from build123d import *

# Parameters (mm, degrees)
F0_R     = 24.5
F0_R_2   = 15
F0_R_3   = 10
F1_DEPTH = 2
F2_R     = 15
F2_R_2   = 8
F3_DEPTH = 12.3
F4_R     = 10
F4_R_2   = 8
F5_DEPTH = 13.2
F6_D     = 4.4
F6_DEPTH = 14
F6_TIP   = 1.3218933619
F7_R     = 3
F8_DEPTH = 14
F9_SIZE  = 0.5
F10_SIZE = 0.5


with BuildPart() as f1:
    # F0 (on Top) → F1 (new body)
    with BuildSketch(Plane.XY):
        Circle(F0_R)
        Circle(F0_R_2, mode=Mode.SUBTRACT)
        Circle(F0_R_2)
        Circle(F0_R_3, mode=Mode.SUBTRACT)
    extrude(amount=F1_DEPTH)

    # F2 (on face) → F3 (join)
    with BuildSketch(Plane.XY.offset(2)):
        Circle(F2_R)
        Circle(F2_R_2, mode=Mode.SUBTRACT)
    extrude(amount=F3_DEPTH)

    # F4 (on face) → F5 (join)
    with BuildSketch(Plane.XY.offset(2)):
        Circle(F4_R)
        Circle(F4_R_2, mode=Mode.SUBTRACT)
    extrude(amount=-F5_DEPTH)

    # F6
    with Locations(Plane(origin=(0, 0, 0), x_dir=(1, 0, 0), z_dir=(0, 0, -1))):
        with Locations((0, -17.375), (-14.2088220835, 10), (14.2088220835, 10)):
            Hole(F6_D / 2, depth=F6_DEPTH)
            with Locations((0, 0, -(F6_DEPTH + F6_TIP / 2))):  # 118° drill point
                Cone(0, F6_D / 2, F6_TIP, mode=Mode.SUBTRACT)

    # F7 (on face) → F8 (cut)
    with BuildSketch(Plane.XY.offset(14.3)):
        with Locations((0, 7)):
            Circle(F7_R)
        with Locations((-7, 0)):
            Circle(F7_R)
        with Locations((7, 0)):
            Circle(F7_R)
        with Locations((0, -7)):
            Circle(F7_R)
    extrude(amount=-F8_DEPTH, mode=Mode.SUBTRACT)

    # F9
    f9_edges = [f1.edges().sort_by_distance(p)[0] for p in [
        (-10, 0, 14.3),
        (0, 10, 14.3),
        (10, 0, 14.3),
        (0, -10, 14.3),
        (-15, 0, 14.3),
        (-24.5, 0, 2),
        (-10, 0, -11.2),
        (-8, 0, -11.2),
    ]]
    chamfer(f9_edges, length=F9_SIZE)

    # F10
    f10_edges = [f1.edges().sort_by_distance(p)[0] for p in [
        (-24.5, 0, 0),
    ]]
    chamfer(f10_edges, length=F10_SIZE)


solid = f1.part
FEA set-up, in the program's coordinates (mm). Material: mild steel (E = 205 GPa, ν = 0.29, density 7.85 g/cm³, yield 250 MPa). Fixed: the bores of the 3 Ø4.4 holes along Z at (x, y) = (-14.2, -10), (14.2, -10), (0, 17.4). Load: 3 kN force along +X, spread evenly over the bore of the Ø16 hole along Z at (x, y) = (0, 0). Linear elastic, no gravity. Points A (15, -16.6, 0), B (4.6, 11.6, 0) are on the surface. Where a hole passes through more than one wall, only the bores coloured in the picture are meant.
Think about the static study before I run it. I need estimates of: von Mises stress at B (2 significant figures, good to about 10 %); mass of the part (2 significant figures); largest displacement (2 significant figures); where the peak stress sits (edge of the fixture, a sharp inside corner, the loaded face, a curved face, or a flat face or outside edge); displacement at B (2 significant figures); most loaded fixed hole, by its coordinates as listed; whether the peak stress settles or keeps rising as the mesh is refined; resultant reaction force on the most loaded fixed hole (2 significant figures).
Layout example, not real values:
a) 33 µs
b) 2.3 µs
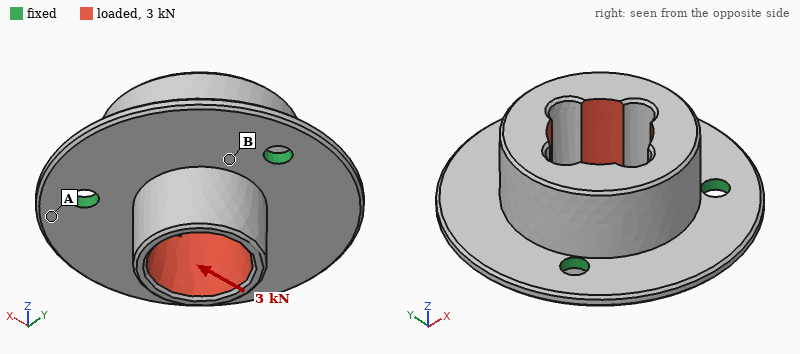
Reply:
a) 23 MPa
b) 80 g
c) 6.9 µm
d) edge of the fixture
e) 1.7 µm
f) (0, 17.4)
g) keeps rising
h) 1.2 kN
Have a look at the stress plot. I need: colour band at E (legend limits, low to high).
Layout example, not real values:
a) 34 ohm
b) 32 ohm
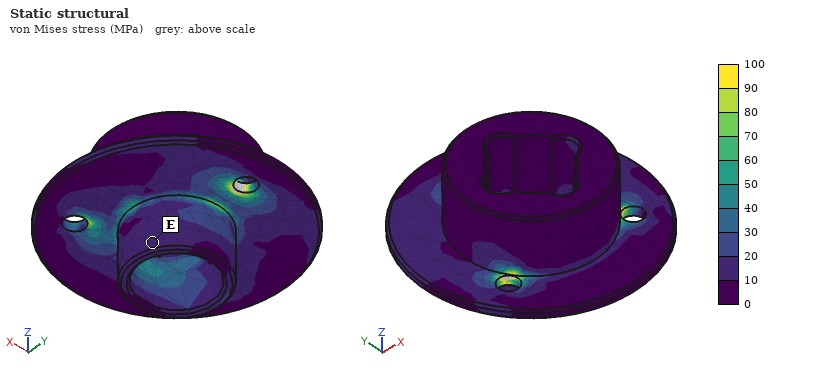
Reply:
a) 10 to 20 MPa
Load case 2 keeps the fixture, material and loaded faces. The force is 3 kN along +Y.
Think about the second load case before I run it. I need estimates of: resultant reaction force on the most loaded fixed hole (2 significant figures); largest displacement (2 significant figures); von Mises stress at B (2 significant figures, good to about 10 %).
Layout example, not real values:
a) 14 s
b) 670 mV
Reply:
a) 1.1 kN
b) 6.8 µm
c) 32 MPa
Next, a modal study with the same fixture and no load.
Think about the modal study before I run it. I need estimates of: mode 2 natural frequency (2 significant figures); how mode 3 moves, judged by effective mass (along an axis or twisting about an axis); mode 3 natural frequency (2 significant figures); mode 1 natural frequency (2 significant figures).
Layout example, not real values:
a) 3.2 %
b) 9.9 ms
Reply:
a) 13 kHz
b) along Z
c) 15 kHz
d) 12 kHz
